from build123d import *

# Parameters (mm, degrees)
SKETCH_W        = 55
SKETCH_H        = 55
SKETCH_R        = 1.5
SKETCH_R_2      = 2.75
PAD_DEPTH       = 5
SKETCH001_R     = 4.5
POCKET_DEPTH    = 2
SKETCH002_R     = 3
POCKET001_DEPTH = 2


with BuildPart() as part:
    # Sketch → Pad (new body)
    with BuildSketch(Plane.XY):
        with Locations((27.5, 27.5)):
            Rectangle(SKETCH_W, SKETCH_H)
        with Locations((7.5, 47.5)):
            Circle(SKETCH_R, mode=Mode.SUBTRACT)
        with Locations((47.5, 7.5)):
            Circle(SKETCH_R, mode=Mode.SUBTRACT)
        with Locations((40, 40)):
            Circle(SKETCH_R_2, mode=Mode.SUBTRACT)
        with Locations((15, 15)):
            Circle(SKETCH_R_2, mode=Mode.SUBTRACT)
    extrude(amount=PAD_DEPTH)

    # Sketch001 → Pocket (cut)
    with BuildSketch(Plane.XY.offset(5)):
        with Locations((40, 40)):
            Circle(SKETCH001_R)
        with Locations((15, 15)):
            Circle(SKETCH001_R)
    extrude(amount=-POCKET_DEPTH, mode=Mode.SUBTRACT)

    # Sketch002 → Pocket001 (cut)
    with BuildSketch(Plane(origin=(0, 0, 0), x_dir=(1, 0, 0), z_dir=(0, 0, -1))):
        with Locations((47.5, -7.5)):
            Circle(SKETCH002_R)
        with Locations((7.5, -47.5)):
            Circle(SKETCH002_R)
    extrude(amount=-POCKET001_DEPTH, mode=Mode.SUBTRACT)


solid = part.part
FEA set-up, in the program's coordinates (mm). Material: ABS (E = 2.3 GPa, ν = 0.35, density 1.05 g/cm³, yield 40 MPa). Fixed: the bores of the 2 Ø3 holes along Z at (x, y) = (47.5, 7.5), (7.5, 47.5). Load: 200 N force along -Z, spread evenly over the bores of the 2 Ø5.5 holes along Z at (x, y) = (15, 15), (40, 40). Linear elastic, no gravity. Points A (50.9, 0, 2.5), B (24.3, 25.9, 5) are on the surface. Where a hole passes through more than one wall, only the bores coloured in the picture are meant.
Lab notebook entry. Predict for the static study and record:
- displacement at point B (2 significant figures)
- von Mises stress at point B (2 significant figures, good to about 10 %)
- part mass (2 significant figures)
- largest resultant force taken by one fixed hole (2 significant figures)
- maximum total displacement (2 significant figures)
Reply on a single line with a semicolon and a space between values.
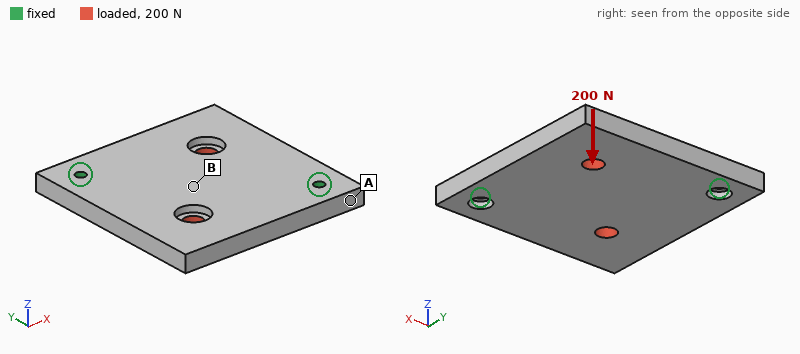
0.40 mm; 8.9 MPa; 15 g; 160 N; 0.86 mm
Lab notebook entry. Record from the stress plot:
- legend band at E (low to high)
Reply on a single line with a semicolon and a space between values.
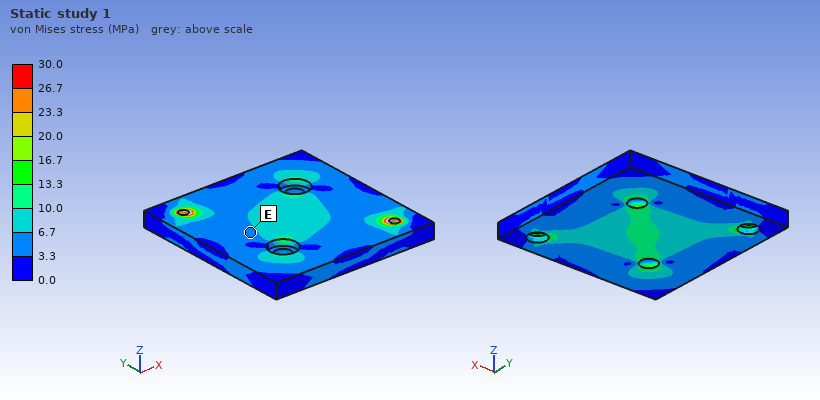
3.3 to 6.7 MPa
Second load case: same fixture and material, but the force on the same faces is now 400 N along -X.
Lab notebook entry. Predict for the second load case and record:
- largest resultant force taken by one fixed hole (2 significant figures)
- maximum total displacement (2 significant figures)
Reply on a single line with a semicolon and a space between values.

200 N; 0.36 mm
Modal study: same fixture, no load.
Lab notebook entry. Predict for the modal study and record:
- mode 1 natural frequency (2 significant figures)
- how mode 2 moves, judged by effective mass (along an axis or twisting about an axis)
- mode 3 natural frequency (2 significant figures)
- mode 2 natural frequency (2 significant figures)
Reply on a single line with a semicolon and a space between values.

620 Hz; along Z; 2600 Hz; 980 Hz
